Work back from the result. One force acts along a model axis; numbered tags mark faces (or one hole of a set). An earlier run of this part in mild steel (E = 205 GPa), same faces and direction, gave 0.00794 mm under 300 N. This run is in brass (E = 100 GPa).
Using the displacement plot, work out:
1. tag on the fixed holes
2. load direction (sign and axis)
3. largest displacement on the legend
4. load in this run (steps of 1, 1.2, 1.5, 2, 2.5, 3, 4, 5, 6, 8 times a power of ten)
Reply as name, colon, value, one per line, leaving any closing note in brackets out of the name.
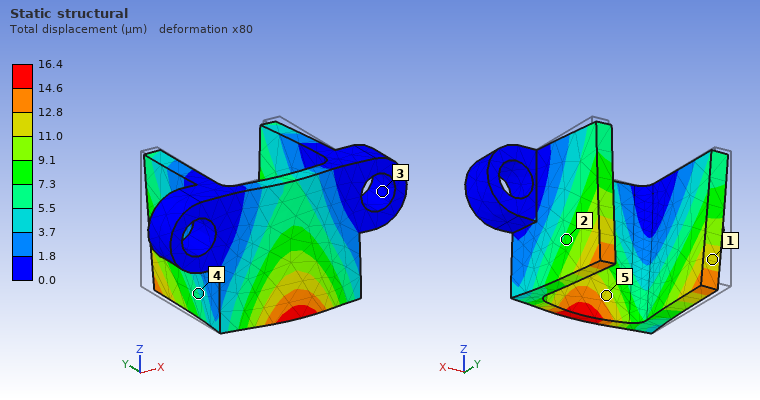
tag on the fixed holes: 3
load direction: -Y
largest displacement on the legend: 16.4 µm
load in this run: 300 N
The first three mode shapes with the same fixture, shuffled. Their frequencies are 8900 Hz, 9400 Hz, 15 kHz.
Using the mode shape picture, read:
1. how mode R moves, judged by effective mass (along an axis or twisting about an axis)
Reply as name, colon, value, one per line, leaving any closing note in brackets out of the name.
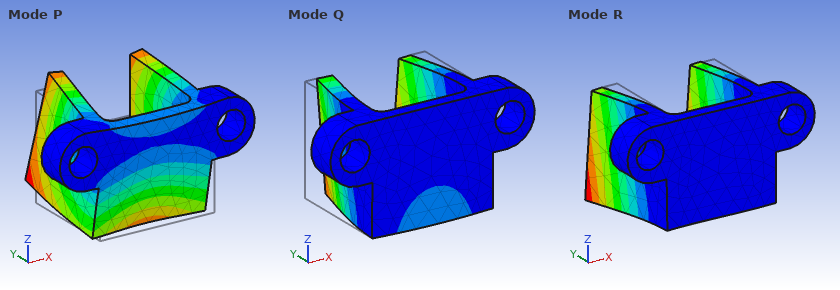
how mode R moves, judged by effective mass: along X
